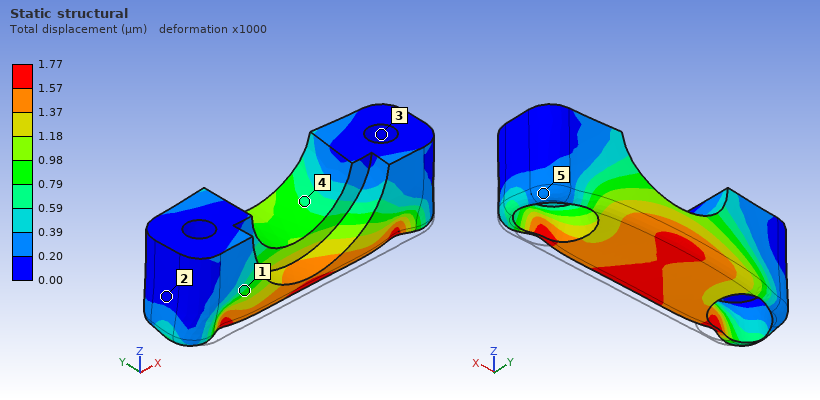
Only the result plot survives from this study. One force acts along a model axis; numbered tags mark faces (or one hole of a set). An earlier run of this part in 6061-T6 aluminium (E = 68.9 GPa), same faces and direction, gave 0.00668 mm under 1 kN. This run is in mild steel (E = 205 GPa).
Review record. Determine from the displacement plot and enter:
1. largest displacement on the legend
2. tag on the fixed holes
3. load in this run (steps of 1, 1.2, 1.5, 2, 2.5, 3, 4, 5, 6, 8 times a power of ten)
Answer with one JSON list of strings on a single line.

["1.77 µm", "3", "800 N"]
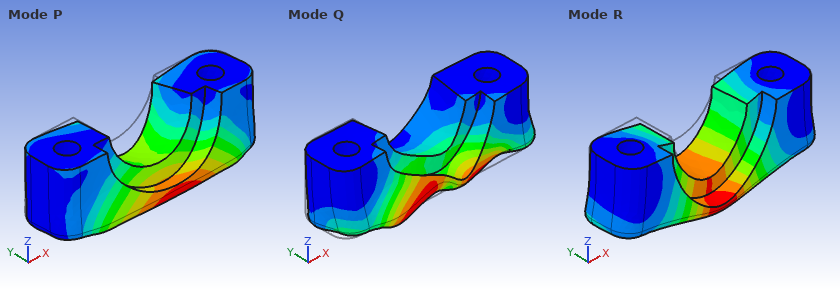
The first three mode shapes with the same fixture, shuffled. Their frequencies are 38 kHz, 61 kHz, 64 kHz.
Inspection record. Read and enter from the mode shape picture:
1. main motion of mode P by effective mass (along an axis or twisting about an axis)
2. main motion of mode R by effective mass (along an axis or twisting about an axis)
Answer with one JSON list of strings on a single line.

["along Y", "along Z"]
